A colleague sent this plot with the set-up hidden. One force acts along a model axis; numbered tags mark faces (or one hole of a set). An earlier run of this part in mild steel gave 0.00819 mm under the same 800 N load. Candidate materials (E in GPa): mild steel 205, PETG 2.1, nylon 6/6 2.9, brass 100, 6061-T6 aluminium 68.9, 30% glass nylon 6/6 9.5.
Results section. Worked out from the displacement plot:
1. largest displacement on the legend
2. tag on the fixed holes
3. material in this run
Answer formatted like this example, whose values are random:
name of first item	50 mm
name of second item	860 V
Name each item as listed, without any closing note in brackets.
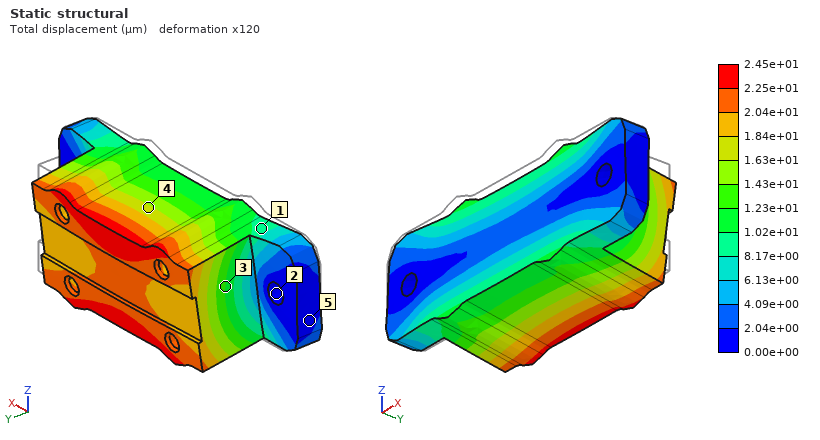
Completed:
largest displacement on the legend	2.45e+01 µm
tag on the fixed holes	2
material in this run	6061-T6 aluminium
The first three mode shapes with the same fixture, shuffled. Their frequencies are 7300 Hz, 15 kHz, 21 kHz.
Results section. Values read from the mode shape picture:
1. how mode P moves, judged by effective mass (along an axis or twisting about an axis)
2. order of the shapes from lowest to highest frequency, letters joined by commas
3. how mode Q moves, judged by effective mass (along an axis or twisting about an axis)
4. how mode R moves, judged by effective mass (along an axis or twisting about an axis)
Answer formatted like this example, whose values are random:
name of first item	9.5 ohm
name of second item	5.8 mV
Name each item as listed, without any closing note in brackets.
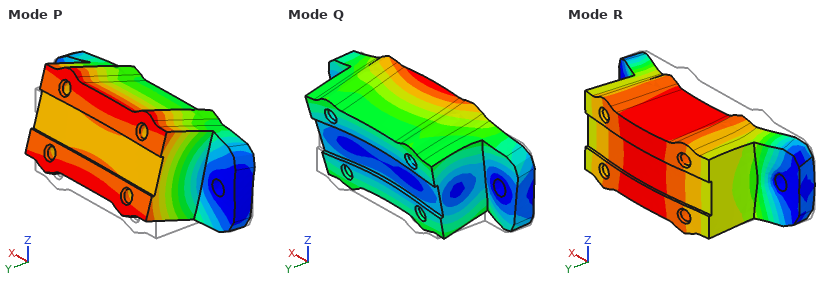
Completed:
how mode P moves, judged by effective mass	along Z
order of the shapes from lowest to highest frequency, letters joined by commas	P, R, Q
how mode Q moves, judged by effective mass	along Z
how mode R moves, judged by effective mass	along Y
